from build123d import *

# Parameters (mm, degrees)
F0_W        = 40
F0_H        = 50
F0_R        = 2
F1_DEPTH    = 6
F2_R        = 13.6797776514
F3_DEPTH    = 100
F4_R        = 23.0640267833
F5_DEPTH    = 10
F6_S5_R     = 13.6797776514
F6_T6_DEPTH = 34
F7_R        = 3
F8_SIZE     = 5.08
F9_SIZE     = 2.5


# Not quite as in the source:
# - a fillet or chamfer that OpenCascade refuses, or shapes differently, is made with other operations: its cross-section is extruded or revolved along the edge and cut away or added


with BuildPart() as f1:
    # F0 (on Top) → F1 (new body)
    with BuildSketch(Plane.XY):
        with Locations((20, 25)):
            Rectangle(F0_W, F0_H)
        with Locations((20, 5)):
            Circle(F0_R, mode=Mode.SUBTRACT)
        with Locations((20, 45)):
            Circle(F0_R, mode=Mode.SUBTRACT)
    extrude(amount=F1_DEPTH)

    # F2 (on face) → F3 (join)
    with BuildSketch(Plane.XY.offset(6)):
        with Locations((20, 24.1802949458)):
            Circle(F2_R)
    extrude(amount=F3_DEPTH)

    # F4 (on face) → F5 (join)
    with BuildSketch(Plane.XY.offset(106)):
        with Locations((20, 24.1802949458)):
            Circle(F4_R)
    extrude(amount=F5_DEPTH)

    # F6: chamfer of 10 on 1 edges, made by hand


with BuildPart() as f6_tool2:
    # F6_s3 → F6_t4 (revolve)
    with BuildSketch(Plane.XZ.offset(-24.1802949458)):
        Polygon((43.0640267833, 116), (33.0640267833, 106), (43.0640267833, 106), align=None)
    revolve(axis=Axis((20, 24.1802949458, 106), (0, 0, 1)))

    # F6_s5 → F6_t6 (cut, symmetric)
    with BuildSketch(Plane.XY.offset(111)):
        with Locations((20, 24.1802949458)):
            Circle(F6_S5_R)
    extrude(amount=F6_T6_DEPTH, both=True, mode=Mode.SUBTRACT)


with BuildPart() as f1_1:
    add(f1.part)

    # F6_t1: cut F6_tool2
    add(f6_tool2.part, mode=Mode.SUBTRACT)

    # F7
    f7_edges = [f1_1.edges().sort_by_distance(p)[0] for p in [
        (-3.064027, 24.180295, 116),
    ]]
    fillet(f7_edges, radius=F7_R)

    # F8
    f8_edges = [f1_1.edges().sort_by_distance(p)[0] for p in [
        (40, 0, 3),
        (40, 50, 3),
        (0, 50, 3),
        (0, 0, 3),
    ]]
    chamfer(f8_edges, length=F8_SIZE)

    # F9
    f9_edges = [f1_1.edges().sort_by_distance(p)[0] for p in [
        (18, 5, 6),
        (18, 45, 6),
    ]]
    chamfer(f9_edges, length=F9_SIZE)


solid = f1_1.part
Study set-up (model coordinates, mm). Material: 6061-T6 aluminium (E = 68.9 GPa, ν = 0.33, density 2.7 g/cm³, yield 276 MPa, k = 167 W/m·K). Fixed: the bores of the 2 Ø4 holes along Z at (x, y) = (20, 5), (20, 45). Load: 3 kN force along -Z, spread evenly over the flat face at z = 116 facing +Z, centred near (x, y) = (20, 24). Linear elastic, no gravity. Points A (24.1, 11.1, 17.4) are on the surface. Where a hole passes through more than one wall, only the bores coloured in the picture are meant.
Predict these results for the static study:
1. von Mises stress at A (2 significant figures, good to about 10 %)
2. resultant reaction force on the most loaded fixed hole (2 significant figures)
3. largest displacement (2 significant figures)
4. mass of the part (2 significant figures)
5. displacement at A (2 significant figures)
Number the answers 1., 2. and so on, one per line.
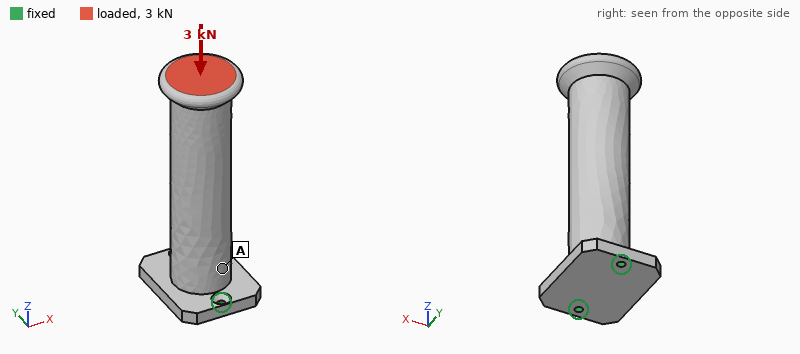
1. 7.6 MPa
2. 1.8 kN
3. 26 µm
4. 210 g
5. 14 µm
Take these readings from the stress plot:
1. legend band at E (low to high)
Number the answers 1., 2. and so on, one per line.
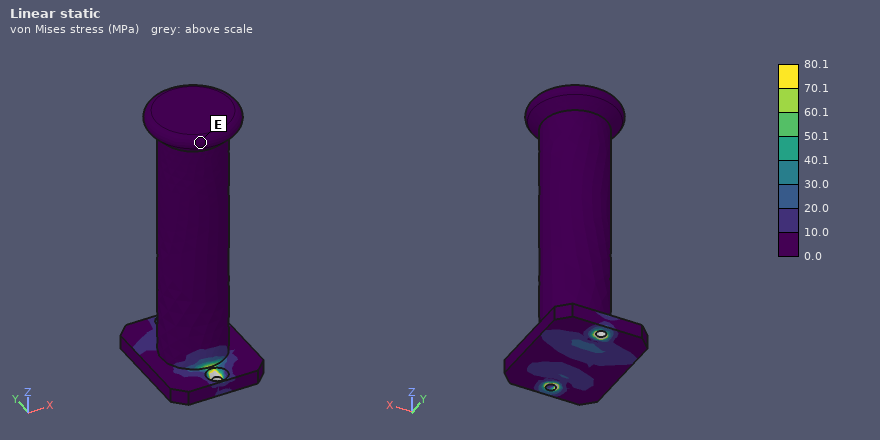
1. 0.0 to 10.0 MPa
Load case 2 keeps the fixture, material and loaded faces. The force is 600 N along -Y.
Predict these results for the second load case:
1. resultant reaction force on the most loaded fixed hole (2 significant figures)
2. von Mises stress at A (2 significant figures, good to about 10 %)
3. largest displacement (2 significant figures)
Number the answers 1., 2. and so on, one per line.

1. 1.9 kN
2. 28 MPa
3. 0.26 mm
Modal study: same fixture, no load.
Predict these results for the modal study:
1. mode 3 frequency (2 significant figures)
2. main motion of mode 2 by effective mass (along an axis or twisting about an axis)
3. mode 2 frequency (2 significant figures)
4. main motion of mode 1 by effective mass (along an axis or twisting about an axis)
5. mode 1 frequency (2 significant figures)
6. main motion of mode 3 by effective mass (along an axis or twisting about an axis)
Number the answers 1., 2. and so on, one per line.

1. 4700 Hz
2. along Y
3. 1000 Hz
4. along X
5. 360 Hz
6. along Z
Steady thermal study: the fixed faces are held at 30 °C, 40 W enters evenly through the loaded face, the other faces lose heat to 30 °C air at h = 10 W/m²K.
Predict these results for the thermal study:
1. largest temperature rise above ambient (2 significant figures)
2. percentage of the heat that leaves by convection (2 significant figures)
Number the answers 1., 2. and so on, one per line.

1. 52 K
2. 9.0 %
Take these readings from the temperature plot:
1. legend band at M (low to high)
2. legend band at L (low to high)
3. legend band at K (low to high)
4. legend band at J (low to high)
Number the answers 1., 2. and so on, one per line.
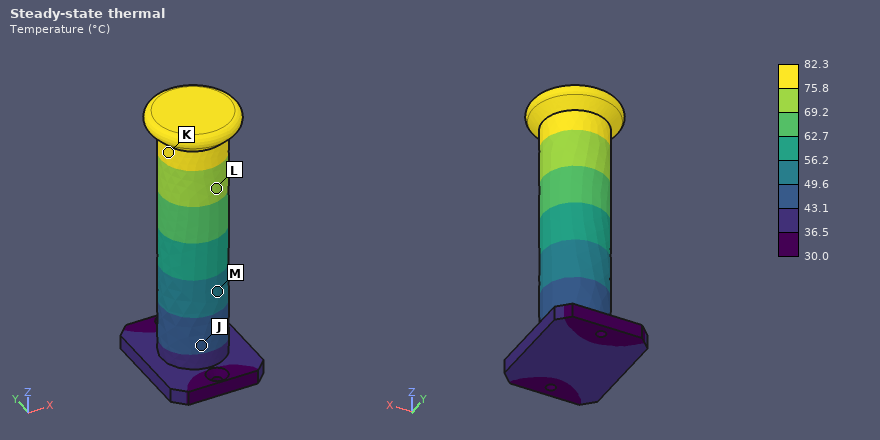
1. 49.6 to 56.2 °C
2. 69.2 to 75.8 °C
3. 75.8 to 82.3 °C
4. 43.1 to 49.6 °C
